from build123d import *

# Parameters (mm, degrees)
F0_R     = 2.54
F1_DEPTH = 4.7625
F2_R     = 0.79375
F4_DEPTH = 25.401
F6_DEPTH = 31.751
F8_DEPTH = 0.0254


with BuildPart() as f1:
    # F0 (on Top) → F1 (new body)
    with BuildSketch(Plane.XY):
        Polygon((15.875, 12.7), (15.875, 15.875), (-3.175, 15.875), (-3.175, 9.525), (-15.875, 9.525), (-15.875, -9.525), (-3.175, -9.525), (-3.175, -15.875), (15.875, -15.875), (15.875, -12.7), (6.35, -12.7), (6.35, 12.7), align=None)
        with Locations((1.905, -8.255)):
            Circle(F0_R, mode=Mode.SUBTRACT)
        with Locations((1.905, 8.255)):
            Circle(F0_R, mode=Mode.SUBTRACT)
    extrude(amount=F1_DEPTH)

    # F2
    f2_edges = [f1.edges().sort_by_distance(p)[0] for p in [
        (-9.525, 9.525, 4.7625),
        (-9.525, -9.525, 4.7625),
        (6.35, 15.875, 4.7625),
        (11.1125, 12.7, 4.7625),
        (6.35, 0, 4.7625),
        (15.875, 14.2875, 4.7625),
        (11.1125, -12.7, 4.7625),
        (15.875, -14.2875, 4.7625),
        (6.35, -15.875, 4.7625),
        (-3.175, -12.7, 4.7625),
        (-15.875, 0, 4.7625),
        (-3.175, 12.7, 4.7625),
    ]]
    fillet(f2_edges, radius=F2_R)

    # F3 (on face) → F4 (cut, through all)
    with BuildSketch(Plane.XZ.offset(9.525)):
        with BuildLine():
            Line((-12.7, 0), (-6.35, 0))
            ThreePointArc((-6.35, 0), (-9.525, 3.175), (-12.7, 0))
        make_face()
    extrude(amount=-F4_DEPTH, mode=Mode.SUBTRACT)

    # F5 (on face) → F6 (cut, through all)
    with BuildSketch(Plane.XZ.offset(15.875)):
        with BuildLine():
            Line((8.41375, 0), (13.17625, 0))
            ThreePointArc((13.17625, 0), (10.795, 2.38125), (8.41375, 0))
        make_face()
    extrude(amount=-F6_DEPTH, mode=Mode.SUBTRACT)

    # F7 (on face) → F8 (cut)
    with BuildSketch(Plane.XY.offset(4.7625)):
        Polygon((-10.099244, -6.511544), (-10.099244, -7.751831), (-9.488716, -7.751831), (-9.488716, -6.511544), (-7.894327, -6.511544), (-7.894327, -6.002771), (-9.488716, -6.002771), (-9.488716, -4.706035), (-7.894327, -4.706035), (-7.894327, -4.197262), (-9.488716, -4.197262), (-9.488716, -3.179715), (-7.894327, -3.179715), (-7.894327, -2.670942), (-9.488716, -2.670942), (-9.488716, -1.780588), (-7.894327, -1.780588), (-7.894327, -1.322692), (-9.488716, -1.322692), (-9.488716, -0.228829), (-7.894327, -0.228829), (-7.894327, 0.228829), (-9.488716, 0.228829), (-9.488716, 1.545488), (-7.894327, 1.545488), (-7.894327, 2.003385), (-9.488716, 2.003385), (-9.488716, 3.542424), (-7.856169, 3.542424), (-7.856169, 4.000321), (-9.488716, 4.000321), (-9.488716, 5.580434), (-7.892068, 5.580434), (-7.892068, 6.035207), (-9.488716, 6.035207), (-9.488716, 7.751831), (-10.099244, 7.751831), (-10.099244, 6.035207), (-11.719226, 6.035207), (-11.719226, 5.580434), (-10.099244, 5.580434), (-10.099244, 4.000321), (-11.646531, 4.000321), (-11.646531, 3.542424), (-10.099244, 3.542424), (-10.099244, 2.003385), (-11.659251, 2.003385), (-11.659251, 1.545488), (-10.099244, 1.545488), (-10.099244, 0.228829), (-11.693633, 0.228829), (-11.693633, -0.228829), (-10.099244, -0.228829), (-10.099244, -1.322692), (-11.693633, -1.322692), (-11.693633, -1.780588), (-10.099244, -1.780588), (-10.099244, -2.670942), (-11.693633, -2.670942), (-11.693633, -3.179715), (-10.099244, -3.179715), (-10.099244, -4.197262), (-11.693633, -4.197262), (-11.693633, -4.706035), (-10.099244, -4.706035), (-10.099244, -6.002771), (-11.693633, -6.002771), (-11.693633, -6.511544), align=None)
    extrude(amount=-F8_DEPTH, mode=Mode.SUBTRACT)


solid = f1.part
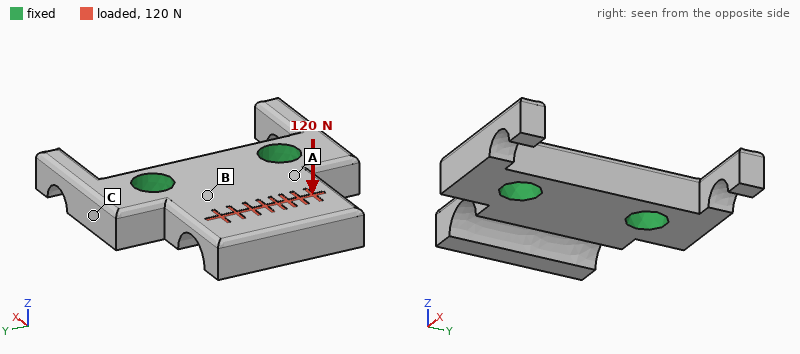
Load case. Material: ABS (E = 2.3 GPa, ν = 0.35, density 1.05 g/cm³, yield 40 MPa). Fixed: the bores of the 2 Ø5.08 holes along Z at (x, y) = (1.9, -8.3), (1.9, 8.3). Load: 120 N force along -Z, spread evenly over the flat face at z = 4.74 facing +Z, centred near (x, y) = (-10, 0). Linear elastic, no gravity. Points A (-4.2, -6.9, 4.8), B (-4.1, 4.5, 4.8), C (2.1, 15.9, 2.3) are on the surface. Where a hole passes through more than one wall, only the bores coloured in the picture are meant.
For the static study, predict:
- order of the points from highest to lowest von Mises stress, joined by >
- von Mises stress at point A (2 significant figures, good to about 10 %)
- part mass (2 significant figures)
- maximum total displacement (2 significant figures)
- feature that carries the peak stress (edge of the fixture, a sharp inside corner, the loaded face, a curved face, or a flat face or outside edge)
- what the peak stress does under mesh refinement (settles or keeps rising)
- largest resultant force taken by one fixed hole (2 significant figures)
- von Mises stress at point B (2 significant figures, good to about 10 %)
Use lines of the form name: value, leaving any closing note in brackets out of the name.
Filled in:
order of the points from highest to lowest von Mises stress, joined by >: A > B > C
von Mises stress at point A: 13 MPa
part mass: 2.4 g
maximum total displacement: 0.46 mm
feature that carries the peak stress: a sharp inside corner
what the peak stress does under mesh refinement: keeps rising
largest resultant force taken by one fixed hole: 63 N
von Mises stress at point B: 9.9 MPa
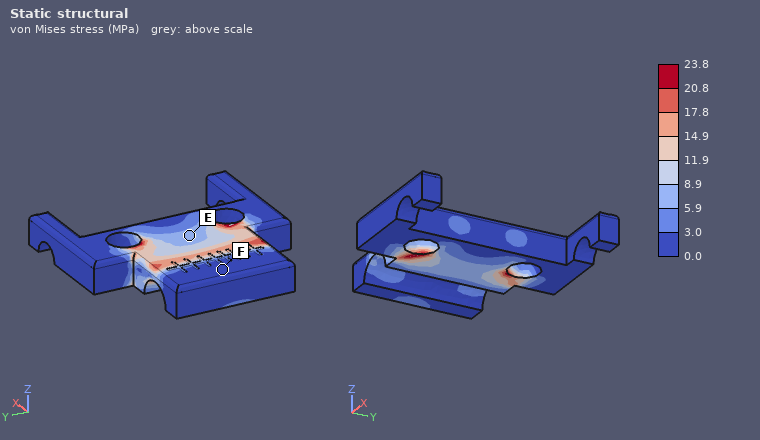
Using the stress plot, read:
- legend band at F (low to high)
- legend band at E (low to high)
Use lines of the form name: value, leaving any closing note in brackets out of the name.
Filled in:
legend band at F: 0.0 to 3.0 MPa
legend band at E: 5.9 to 8.9 MPa
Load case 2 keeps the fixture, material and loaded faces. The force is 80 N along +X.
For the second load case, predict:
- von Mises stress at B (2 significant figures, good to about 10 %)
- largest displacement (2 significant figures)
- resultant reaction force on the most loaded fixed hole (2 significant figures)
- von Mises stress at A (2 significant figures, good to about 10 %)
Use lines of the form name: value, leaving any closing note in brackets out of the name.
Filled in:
von Mises stress at B: 3.5 MPa
largest displacement: 0.13 mm
resultant reaction force on the most loaded fixed hole: 44 N
von Mises stress at A: 4.3 MPa
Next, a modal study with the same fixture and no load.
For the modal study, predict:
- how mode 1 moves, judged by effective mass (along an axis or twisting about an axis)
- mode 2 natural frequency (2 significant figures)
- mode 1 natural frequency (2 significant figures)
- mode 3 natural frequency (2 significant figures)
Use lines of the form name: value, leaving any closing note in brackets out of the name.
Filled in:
how mode 1 moves, judged by effective mass: along Z
mode 2 natural frequency: 5100 Hz
mode 1 natural frequency: 2700 Hz
mode 3 natural frequency: 5100 Hz
